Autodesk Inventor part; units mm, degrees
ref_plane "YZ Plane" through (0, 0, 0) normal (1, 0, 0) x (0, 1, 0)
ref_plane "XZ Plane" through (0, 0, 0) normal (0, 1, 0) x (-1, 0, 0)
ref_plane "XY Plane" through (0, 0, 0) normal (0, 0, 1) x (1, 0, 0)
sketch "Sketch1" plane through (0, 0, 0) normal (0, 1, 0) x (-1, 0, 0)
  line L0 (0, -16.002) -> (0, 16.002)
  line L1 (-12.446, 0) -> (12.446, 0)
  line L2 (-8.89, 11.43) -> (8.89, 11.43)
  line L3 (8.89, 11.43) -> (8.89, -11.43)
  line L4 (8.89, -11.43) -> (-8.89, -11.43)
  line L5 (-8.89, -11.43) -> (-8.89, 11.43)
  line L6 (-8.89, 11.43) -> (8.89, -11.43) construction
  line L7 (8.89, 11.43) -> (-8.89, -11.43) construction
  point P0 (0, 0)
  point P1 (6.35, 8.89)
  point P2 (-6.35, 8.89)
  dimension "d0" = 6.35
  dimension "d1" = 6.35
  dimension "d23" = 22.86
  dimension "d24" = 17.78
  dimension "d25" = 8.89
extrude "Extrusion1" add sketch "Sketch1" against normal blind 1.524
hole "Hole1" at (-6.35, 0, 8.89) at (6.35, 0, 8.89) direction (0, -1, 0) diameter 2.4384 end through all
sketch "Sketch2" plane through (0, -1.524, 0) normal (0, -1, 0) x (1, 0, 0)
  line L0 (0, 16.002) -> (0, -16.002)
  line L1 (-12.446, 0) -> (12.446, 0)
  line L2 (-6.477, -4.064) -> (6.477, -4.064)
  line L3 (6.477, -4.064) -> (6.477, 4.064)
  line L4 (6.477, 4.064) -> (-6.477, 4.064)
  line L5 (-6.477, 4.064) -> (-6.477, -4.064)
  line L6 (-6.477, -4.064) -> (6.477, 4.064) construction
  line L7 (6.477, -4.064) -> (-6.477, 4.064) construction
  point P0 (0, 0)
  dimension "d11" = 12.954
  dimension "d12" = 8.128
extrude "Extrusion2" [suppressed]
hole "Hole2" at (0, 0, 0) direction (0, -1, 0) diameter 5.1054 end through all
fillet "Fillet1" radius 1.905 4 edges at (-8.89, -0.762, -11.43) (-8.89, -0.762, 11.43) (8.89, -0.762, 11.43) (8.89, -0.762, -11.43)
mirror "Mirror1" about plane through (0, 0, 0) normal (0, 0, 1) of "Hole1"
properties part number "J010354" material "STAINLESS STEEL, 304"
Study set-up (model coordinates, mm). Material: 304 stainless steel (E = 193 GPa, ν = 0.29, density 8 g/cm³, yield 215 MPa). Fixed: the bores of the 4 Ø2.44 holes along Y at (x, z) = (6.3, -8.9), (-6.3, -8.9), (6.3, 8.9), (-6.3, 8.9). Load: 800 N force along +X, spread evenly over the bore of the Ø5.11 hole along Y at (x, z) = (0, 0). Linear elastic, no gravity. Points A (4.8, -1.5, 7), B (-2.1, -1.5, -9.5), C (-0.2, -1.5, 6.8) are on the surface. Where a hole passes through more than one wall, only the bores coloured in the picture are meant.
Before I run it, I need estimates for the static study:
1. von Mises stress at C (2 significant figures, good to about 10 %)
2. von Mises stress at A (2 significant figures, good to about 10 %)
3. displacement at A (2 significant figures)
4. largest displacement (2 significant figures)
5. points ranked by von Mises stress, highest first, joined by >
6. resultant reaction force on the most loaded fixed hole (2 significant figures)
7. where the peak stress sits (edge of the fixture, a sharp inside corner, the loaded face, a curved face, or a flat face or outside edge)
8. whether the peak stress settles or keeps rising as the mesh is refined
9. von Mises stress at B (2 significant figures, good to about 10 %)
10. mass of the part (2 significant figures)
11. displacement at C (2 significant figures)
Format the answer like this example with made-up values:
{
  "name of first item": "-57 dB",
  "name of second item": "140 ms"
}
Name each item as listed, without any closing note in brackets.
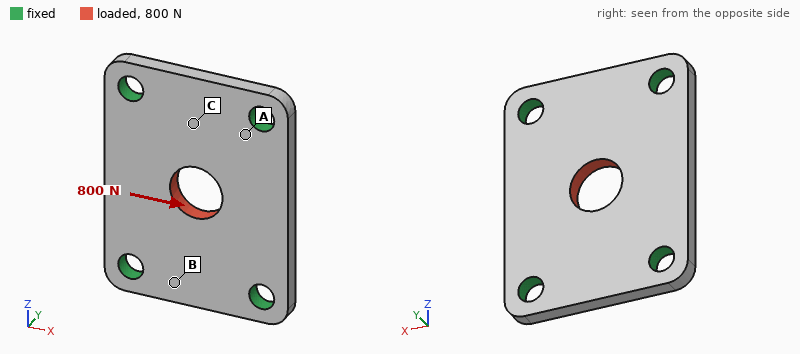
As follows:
{
  "von Mises stress at C": "23 MPa",
  "von Mises stress at A": "36 MPa",
  "displacement at A": "0.35 µm",
  "largest displacement": "2.1 µm",
  "points ranked by von Mises stress, highest first, joined by >": "A > C > B",
  "resultant reaction force on the most loaded fixed hole": "230 N",
  "where the peak stress sits": "edge of the fixture",
  "whether the peak stress settles or keeps rising as the mesh is refined": "keeps rising",
  "von Mises stress at B": "9.2 MPa",
  "mass of the part": "4.4 g",
  "displacement at C": "0.57 µm"
}
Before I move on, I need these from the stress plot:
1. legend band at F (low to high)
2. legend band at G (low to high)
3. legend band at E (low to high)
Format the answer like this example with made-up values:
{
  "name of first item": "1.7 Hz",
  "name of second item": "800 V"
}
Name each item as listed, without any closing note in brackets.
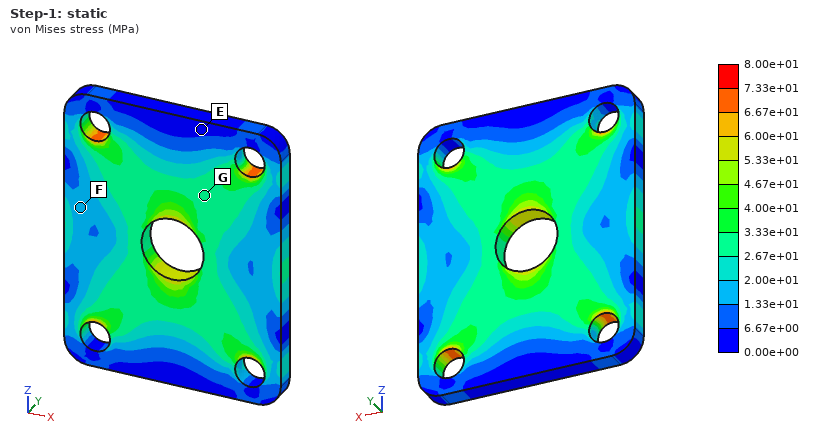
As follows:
{
  "legend band at F": "1.33e+01 to 2.00e+01 MPa",
  "legend band at G": "2.67e+01 to 3.33e+01 MPa",
  "legend band at E": "0.00e+00 to 6.67e+00 MPa"
}
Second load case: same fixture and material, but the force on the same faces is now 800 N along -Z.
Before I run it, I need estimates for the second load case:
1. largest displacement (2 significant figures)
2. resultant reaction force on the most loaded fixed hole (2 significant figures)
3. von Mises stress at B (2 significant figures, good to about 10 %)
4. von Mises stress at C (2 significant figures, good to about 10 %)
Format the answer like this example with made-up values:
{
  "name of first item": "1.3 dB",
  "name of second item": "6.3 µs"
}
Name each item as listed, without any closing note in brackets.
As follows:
{
  "largest displacement": "1.3 µm",
  "resultant reaction force on the most loaded fixed hole": "210 N",
  "von Mises stress at B": "9.6 MPa",
  "von Mises stress at C": "11 MPa"
}
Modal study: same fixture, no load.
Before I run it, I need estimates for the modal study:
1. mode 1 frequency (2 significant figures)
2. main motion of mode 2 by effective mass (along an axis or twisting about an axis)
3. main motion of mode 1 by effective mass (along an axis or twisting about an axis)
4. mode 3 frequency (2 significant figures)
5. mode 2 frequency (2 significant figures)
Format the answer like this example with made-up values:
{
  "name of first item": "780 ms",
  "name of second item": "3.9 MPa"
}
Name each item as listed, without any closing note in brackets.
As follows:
{
  "mode 1 frequency": "25 kHz",
  "main motion of mode 2 by effective mass": "twisting about Z",
  "main motion of mode 1 by effective mass": "along Y",
  "mode 3 frequency": "42 kHz",
  "mode 2 frequency": "32 kHz"
}
